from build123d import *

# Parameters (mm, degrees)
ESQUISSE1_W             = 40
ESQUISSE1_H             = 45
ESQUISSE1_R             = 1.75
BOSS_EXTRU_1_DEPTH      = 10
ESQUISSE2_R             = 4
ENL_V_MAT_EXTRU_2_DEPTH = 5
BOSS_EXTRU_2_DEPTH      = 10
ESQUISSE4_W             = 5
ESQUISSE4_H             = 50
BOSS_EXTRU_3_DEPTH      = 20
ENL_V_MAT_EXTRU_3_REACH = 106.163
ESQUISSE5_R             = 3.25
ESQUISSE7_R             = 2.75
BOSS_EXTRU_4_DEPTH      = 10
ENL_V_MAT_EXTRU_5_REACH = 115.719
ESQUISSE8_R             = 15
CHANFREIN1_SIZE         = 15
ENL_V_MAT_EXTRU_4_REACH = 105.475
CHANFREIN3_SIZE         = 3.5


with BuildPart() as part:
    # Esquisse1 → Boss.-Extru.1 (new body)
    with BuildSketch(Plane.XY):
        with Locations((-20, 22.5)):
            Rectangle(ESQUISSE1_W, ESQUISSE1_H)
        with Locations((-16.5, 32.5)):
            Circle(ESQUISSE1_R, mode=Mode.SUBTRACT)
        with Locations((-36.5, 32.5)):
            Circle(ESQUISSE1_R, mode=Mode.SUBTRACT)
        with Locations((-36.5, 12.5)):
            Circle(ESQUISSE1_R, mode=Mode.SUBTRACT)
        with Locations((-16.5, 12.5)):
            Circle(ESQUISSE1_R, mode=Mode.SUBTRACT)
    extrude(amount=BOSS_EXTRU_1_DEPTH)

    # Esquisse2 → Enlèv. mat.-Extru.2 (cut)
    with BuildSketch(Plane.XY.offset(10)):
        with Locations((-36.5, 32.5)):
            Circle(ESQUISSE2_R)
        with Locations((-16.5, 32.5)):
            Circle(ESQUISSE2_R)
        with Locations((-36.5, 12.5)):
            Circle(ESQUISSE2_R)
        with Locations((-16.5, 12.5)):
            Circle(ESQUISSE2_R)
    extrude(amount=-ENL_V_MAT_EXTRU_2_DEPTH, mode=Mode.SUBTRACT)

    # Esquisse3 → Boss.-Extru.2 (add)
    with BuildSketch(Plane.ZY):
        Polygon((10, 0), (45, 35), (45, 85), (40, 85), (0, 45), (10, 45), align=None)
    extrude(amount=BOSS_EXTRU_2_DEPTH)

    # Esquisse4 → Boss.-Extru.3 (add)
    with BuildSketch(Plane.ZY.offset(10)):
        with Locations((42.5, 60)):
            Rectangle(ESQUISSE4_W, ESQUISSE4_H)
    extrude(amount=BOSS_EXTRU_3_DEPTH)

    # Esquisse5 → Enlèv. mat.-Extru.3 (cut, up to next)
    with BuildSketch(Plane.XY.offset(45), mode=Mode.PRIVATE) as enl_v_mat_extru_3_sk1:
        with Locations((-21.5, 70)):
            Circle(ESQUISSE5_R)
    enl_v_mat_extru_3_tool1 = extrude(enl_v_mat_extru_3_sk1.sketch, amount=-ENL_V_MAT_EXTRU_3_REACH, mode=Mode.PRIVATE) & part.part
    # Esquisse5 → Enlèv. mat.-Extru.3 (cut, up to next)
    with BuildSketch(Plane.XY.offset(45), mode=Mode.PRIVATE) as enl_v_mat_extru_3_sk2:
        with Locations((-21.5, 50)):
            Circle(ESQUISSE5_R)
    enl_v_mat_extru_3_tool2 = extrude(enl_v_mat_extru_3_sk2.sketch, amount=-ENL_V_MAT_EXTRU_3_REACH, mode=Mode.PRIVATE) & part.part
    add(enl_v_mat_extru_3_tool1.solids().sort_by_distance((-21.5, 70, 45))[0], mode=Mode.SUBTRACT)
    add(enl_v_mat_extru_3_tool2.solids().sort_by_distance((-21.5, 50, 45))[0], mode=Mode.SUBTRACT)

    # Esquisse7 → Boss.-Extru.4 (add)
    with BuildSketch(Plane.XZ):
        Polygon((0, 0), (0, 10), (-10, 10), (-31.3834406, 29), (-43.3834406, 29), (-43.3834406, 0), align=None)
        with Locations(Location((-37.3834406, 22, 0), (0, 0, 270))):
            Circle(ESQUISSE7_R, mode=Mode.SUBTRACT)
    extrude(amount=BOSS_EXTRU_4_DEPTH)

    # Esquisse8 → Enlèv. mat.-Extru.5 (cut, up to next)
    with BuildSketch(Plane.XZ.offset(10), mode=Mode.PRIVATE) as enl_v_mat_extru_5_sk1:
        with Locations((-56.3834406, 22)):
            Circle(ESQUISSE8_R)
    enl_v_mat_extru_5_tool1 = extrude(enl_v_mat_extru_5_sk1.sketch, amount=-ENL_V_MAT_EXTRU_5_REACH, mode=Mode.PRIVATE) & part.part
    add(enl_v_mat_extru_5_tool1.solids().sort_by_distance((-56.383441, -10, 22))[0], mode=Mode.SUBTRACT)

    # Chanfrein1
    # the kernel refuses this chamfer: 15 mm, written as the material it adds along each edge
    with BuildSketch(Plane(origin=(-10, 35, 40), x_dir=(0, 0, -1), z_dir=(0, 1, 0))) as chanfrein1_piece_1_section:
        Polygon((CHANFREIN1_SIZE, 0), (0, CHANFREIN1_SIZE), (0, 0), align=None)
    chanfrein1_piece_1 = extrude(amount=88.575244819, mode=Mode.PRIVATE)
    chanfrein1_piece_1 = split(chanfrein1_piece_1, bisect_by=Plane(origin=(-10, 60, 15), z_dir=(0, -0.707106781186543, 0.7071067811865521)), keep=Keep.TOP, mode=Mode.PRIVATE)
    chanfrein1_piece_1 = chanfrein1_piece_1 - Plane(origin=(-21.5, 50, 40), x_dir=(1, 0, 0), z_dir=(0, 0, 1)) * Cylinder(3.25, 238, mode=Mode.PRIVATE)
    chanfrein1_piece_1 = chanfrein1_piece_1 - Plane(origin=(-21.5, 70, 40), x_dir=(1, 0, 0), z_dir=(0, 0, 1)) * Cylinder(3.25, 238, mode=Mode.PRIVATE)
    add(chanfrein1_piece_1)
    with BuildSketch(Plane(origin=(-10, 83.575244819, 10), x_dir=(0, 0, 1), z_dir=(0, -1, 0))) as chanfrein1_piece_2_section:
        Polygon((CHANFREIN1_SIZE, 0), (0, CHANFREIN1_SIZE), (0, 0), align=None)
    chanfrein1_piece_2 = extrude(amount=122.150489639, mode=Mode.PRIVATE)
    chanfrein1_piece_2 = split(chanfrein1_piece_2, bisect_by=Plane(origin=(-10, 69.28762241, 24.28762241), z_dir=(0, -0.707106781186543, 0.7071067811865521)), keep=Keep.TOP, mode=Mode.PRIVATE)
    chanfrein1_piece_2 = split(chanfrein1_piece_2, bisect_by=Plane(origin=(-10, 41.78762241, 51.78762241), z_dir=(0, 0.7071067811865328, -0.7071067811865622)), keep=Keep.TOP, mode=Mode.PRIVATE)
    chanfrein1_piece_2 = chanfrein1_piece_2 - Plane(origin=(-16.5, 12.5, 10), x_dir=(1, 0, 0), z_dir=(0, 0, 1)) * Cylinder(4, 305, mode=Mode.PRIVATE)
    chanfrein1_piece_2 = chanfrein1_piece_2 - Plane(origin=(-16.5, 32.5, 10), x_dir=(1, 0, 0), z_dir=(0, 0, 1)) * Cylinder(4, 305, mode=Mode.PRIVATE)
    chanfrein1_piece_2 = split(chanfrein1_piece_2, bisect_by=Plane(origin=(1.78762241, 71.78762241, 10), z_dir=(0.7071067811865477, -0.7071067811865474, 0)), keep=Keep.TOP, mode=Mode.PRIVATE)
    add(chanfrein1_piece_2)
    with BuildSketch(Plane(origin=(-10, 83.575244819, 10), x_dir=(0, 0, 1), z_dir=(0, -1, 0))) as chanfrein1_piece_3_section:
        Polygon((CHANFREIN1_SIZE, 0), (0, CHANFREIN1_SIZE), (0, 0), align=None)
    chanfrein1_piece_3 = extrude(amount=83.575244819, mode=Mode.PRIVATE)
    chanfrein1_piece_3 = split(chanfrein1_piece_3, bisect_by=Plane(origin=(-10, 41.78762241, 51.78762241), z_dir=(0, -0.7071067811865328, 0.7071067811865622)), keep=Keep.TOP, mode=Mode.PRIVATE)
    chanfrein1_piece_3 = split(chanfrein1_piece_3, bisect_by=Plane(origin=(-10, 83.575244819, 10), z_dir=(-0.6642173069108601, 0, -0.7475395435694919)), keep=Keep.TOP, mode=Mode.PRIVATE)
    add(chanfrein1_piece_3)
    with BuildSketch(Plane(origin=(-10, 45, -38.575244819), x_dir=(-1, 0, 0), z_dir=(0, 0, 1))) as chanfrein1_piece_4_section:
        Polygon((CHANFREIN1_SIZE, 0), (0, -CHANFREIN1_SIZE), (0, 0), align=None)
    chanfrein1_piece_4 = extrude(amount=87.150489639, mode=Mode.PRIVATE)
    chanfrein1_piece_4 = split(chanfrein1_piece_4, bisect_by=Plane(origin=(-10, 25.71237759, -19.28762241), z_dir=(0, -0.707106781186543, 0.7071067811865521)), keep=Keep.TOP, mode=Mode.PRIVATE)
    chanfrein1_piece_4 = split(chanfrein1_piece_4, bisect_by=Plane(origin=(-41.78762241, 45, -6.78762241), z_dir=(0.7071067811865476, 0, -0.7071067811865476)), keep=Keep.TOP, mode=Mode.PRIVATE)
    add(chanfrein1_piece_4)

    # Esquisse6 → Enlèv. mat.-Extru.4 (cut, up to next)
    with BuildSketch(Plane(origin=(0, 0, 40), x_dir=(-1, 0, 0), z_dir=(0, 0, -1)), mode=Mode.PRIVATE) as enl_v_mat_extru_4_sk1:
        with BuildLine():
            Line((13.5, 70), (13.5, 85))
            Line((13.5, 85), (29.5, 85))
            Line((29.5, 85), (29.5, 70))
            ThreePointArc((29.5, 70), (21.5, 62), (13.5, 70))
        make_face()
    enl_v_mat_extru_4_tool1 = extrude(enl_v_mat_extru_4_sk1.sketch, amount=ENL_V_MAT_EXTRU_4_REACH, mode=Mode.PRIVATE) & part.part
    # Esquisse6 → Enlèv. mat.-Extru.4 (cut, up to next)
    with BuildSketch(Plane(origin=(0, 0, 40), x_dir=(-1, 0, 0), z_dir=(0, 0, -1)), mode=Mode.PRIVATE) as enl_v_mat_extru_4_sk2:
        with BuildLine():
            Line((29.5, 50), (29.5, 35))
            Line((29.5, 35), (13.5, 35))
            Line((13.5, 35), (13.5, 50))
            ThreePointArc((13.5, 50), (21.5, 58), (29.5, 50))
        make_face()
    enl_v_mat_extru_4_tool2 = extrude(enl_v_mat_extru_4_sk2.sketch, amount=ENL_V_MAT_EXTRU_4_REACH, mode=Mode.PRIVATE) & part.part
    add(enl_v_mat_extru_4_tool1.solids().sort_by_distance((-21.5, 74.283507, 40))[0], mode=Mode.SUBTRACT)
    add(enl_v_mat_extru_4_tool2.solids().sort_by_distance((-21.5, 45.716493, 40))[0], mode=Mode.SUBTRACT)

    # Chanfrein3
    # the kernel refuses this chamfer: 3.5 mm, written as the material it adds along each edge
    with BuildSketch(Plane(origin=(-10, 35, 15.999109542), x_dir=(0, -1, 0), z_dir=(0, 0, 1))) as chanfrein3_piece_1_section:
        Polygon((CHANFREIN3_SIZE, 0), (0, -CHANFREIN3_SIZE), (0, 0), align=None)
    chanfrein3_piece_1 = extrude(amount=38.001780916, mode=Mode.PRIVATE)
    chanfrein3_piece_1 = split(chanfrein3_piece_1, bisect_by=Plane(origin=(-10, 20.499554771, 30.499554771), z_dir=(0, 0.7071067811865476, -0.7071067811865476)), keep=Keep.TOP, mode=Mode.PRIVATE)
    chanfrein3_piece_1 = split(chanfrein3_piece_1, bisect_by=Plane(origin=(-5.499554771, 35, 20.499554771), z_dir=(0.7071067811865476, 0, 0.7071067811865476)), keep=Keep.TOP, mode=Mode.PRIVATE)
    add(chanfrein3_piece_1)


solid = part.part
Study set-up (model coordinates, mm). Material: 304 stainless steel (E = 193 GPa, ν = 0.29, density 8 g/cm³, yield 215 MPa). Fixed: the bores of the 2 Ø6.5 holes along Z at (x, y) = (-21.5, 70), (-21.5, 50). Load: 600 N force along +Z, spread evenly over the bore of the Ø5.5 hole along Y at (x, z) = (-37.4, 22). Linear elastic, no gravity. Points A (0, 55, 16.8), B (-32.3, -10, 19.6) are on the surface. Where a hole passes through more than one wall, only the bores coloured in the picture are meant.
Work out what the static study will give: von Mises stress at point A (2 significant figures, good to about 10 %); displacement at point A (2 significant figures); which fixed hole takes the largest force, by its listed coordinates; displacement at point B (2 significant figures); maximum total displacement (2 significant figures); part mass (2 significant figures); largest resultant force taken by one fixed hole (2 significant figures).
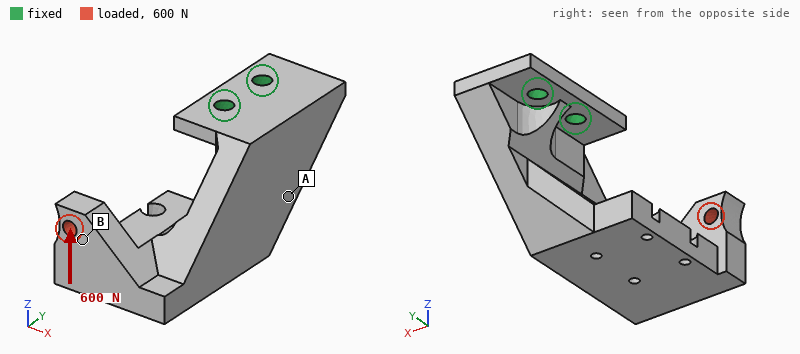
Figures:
19 MPa
25 µm
(-21.5, 50)
72 µm
98 µm
460 g
1.8 kN
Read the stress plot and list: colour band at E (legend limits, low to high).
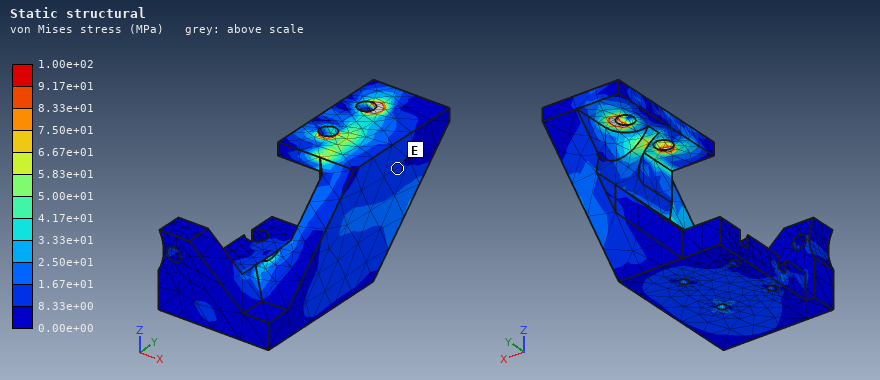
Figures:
8.33e+00 to 1.67e+01 MPa
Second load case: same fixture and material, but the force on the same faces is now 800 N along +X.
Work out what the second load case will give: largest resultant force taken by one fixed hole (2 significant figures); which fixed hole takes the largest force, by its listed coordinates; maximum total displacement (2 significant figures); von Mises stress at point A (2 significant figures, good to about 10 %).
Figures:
2.5 kN
(-21.5, 50)
0.12 mm
31 MPa
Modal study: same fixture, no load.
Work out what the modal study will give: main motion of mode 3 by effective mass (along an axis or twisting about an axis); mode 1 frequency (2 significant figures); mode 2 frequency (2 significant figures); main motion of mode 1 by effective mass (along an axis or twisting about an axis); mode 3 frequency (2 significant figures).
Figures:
along Z
860 Hz
1300 Hz
along X
2700 Hz
